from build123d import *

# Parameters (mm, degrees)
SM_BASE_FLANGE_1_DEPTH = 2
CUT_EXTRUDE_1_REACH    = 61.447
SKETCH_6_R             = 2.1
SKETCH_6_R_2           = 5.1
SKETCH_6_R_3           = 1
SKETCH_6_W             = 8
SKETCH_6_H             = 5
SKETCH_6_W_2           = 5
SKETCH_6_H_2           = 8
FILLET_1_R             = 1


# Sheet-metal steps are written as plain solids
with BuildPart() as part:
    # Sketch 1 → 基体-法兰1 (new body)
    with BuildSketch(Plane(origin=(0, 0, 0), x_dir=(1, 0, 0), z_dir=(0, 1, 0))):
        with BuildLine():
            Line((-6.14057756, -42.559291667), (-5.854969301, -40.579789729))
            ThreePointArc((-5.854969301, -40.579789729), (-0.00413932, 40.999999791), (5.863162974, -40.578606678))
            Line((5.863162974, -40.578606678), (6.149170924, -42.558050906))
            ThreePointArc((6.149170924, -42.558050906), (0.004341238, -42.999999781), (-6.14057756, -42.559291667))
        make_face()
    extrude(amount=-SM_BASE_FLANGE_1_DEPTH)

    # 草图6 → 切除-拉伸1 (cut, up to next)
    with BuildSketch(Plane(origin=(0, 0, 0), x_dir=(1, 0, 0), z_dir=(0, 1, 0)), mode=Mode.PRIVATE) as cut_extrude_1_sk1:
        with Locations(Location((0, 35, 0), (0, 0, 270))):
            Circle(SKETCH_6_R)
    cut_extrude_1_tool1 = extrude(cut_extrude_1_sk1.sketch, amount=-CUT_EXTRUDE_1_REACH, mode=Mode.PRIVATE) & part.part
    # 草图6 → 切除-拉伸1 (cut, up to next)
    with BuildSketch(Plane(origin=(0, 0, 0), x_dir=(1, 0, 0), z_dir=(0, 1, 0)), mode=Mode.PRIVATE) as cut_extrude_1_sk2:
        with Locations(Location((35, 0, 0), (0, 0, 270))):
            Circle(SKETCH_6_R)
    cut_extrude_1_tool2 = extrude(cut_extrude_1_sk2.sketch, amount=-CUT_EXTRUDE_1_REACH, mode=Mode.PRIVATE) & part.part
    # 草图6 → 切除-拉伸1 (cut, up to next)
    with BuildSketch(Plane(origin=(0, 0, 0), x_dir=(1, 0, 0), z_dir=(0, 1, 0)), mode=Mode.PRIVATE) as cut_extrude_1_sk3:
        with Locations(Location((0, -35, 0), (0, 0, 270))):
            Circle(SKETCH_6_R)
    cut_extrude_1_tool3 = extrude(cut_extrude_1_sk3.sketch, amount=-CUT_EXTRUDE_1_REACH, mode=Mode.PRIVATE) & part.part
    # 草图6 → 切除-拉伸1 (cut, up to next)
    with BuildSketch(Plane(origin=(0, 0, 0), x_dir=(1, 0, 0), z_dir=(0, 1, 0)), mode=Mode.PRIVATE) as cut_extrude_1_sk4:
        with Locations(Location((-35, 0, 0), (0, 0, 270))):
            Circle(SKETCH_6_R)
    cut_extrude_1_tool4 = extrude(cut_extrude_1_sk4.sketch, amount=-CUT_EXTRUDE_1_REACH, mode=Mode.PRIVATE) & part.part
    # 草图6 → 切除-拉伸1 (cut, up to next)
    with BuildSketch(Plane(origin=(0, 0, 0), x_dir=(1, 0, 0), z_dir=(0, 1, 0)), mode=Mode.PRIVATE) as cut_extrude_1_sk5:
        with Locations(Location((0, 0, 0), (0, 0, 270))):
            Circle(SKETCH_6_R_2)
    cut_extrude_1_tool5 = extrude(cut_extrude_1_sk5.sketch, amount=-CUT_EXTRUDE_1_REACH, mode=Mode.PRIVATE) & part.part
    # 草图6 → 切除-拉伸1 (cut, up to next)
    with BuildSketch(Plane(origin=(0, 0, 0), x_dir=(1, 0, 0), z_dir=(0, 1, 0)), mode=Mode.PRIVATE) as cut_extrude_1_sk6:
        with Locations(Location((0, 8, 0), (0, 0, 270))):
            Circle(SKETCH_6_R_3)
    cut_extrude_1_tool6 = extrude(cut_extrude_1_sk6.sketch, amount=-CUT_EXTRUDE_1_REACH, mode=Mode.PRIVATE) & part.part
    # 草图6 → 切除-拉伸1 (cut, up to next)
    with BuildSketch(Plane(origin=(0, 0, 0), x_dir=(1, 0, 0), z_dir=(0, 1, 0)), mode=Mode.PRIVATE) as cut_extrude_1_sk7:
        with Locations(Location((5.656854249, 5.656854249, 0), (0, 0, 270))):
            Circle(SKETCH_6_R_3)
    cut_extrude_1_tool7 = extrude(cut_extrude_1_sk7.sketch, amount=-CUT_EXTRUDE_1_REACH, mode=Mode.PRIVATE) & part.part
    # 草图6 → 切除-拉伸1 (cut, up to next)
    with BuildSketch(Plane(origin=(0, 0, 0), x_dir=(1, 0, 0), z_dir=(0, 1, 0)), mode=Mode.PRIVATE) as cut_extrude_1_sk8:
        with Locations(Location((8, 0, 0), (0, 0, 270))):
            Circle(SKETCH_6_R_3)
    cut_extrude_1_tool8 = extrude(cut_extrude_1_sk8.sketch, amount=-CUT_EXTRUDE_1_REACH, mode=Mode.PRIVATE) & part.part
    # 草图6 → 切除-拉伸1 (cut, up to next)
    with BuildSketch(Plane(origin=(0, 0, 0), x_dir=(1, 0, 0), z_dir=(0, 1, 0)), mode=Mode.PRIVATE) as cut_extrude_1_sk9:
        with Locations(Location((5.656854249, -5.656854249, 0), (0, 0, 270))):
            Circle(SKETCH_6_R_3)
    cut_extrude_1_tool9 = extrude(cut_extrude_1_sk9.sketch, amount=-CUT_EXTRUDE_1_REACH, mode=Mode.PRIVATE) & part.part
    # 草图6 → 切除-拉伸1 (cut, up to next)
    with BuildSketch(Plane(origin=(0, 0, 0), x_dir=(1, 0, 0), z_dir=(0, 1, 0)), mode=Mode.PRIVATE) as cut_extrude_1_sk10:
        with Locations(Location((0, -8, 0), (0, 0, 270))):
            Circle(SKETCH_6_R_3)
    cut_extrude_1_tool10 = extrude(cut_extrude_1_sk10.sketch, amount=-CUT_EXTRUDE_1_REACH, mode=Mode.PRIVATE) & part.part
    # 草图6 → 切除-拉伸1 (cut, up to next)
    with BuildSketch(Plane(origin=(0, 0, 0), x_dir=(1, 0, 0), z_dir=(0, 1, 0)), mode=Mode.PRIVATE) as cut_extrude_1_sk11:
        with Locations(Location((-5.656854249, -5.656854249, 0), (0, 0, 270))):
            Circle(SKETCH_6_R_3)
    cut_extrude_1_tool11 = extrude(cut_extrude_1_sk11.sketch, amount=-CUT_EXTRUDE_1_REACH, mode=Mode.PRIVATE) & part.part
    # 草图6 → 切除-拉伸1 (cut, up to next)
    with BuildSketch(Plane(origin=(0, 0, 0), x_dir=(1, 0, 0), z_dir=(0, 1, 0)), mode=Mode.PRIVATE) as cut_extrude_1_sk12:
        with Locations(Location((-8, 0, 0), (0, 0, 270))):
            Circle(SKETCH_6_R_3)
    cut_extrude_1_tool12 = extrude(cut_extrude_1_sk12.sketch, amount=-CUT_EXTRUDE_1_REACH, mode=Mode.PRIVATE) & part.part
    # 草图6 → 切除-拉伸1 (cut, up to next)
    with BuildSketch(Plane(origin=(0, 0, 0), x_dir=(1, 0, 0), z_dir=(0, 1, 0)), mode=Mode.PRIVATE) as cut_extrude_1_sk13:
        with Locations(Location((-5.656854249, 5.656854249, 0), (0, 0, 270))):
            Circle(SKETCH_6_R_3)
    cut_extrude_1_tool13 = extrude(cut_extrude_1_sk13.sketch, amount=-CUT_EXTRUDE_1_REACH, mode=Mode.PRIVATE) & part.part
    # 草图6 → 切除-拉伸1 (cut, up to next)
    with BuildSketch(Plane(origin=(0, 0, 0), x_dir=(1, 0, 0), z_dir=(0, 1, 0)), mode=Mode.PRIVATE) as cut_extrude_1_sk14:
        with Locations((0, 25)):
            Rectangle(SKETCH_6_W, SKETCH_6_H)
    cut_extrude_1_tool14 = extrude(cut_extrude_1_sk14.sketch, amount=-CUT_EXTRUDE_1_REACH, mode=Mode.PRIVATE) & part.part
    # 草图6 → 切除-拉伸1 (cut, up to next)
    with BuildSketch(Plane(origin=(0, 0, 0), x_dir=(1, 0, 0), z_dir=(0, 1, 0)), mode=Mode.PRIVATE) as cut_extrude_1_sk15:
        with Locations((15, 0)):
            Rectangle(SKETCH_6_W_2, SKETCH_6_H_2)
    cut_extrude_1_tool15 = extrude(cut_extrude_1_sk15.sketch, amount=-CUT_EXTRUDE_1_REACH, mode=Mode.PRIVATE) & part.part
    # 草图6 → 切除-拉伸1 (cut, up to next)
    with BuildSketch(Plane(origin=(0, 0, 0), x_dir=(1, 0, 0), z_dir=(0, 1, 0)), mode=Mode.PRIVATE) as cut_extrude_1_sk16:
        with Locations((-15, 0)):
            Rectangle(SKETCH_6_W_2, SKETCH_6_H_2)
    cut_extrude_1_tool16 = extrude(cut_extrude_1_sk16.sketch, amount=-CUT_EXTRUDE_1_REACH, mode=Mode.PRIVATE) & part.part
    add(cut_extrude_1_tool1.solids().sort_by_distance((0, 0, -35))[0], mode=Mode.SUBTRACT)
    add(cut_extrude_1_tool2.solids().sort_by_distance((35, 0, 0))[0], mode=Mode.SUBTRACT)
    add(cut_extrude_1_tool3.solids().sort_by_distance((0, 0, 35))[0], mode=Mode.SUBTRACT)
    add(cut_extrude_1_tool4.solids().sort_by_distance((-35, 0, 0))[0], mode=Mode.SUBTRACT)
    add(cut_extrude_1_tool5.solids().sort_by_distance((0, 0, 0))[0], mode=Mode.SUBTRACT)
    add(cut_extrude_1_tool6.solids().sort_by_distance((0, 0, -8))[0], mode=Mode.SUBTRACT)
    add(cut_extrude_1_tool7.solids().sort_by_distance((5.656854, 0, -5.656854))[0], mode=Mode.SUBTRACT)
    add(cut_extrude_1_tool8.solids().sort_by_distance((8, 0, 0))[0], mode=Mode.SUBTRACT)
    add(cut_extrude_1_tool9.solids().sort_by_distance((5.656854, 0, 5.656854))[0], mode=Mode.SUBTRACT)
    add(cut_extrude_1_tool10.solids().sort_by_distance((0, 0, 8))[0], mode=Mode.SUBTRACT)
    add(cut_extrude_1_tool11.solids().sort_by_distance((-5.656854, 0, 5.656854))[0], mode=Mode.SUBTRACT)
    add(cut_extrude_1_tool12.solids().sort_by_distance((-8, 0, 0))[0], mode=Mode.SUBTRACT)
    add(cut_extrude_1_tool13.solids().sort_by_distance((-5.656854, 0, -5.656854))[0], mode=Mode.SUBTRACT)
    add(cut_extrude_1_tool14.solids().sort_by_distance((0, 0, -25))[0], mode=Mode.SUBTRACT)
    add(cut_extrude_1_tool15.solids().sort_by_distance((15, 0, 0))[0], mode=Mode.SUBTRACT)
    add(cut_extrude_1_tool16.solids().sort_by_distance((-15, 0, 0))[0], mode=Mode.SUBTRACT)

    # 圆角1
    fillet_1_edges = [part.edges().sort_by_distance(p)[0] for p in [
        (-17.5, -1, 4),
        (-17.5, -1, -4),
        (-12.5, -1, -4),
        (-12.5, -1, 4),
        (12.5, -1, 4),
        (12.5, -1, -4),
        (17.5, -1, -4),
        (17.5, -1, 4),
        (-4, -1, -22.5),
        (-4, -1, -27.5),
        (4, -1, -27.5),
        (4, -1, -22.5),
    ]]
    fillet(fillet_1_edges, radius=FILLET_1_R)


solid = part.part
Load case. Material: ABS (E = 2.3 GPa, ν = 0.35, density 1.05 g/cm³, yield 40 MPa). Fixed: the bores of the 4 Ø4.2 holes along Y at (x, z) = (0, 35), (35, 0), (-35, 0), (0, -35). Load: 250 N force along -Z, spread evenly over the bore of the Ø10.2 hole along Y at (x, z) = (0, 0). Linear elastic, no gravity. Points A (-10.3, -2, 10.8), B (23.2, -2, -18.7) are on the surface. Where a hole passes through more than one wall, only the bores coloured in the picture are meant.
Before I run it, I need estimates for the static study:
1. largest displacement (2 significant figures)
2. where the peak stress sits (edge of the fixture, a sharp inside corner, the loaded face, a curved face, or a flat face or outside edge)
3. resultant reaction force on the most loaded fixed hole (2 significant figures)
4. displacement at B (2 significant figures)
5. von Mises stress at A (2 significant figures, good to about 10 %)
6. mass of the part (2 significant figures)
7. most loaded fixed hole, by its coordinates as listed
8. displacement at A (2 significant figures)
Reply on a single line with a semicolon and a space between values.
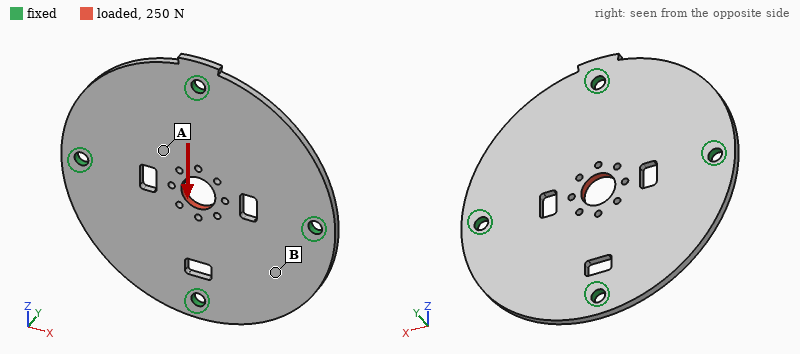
49 µm; a curved face; 91 N; 17 µm; 1.9 MPa; 11 g; (0, 35); 26 µm
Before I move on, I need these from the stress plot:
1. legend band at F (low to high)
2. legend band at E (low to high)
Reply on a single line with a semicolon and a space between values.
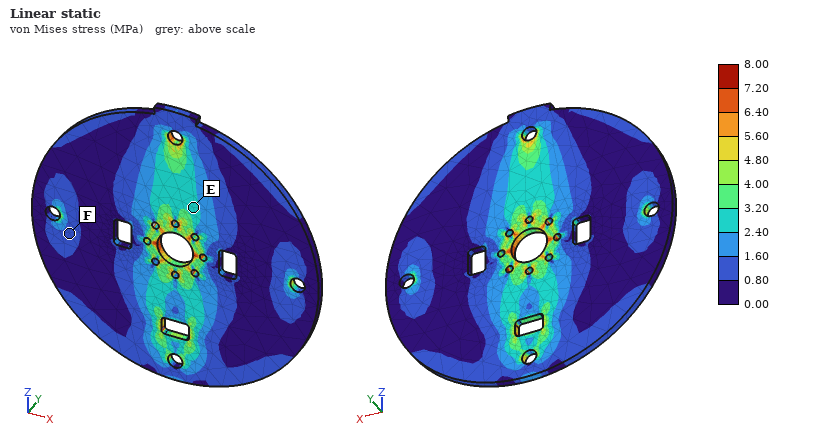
0.80 to 1.60 MPa; 2.40 to 3.20 MPa
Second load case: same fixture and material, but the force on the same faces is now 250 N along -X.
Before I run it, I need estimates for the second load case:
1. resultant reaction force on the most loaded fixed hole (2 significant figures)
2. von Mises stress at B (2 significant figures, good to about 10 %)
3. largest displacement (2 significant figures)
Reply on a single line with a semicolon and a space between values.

77 N; 0.76 MPa; 54 µm
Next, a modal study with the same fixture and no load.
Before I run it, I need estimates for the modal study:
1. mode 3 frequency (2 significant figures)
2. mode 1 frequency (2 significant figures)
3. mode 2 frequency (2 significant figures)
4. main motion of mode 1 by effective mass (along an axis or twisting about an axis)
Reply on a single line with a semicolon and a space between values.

1100 Hz; 930 Hz; 1100 Hz; along Y
